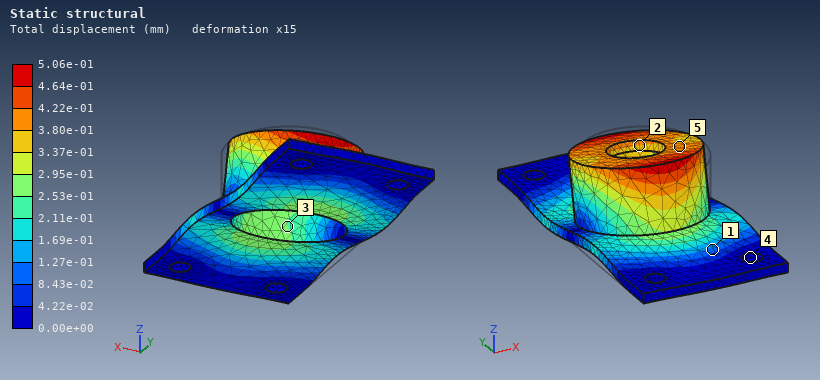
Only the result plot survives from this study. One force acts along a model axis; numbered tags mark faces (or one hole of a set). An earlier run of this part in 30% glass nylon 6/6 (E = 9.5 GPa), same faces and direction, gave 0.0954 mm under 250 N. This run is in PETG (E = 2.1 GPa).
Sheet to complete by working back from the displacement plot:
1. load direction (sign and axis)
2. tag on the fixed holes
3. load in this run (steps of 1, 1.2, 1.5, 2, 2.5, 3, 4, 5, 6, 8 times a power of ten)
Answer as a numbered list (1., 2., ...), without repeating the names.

1. +Y
2. 4
3. 300 N
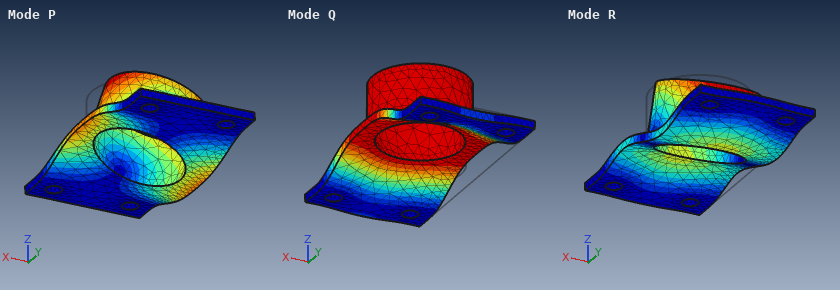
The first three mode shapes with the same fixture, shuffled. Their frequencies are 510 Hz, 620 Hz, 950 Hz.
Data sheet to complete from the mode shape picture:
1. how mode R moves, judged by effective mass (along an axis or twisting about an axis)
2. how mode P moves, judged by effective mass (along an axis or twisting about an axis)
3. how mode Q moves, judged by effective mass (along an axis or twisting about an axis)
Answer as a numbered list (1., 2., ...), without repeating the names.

1. along Y
2. along X
3. along Z
